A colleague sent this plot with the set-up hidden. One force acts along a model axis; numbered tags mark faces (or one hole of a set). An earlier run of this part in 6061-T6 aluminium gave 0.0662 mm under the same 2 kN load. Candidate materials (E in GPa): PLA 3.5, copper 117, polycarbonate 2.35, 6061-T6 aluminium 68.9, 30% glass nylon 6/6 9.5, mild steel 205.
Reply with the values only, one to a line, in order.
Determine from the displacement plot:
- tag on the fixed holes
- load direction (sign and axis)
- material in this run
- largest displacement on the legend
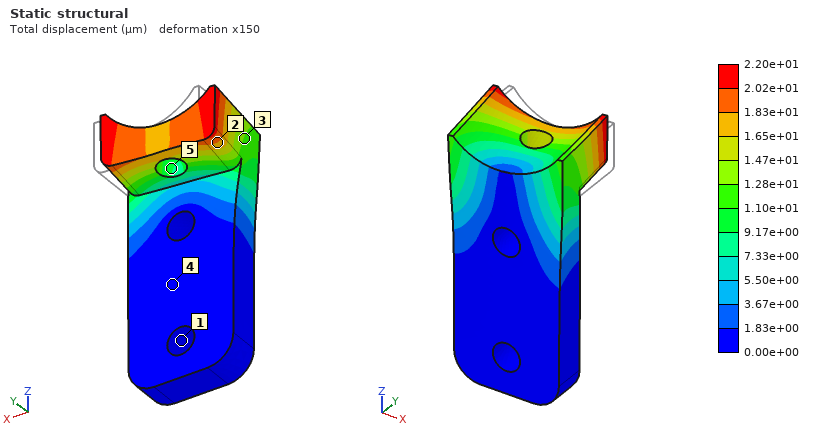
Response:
1
-X
mild steel
2.20e+01 µm
